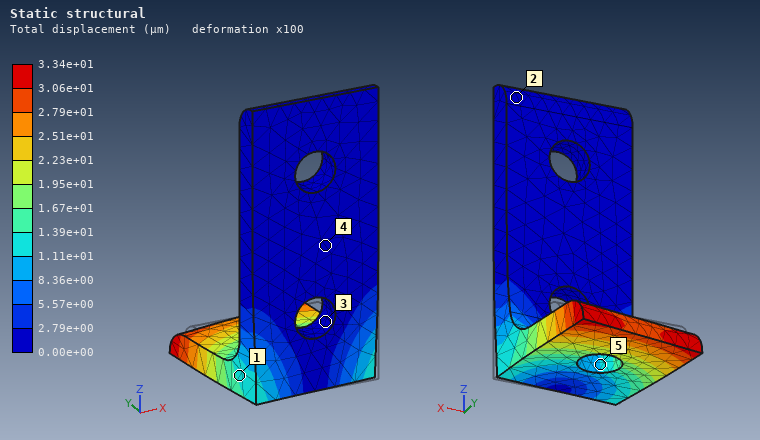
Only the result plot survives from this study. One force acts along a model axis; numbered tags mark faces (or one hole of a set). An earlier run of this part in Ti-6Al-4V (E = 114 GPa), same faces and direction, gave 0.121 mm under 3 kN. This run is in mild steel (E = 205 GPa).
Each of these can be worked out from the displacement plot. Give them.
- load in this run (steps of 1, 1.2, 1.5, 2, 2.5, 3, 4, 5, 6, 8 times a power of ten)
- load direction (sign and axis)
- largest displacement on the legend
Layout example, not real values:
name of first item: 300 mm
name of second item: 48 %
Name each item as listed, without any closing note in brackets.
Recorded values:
load in this run: 1.5 kN
load direction: -X
largest displacement on the legend: 3.34e+01 µm
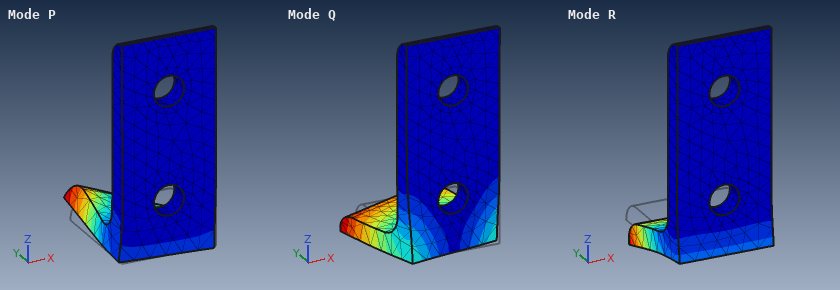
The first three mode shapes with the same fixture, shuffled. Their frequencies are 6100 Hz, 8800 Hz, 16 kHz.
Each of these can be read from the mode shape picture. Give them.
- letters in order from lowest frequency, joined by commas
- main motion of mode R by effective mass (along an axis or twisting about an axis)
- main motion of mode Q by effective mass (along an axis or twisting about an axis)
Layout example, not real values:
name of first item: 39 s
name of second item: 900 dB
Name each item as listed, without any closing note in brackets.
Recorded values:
letters in order from lowest frequency, joined by commas: R, Q, P
main motion of mode R by effective mass: along Z
main motion of mode Q by effective mass: along X
